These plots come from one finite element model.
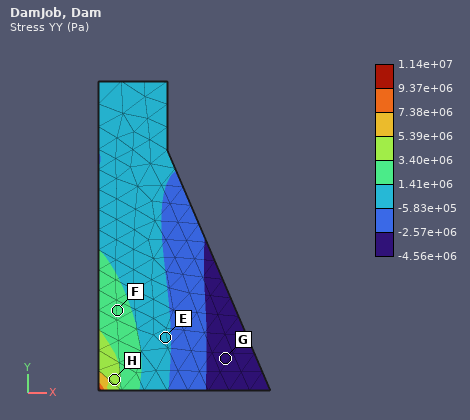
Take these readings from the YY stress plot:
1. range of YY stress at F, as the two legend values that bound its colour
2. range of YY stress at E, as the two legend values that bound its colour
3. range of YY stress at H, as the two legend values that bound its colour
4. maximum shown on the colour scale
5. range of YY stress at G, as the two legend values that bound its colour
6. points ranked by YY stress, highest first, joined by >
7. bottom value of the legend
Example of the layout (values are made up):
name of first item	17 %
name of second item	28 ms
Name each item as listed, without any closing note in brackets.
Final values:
range of YY stress at F, as the two legend values that bound its colour	1.41e+06 to 3.40e+06 Pa
range of YY stress at E, as the two legend values that bound its colour	-5.83e+05 to 1.41e+06 Pa
range of YY stress at H, as the two legend values that bound its colour	3.40e+06 to 5.39e+06 Pa
maximum shown on the colour scale	1.14e+07 Pa
range of YY stress at G, as the two legend values that bound its colour	-4.56e+06 to -2.57e+06 Pa
points ranked by YY stress, highest first, joined by >	H > F > E > G
bottom value of the legend	-4.56e+06 Pa
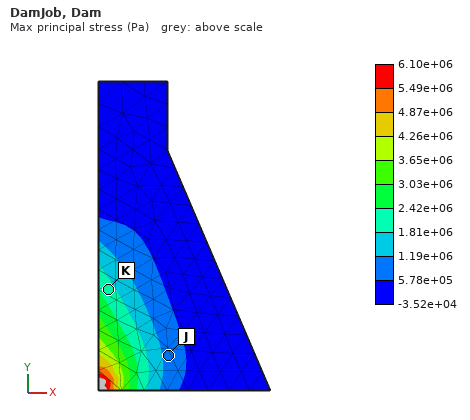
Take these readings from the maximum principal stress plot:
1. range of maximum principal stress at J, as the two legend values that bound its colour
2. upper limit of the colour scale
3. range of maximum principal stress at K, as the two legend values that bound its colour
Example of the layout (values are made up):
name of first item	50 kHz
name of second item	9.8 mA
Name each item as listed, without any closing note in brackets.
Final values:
range of maximum principal stress at J, as the two legend values that bound its colour	5.78e+05 to 1.19e+06 Pa
upper limit of the colour scale	6.10e+06 Pa
range of maximum principal stress at K, as the two legend values that bound its colour	1.81e+06 to 2.42e+06 Pa
